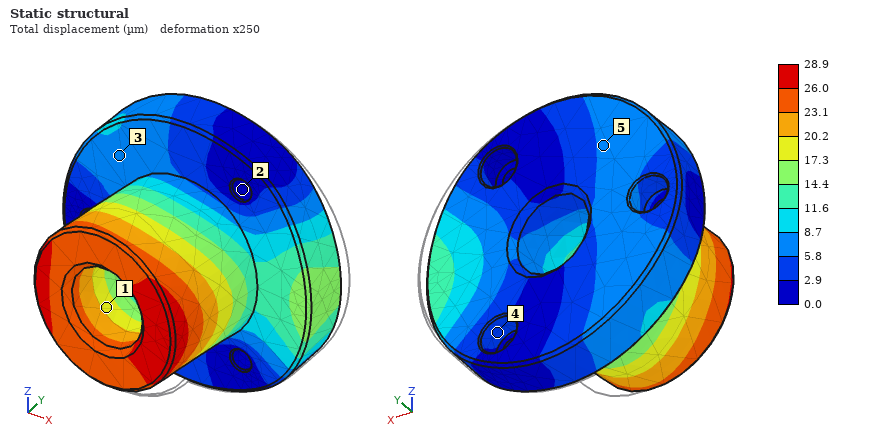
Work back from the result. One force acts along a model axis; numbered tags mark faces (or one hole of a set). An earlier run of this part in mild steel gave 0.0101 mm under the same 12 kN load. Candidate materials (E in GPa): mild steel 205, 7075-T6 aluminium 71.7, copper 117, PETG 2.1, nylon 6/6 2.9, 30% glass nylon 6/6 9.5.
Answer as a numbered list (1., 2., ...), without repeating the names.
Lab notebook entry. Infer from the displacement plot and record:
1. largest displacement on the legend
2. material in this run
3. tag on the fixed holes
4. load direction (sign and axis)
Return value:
1. 28.9 µm
2. 7075-T6 aluminium
3. 2
4. -X
